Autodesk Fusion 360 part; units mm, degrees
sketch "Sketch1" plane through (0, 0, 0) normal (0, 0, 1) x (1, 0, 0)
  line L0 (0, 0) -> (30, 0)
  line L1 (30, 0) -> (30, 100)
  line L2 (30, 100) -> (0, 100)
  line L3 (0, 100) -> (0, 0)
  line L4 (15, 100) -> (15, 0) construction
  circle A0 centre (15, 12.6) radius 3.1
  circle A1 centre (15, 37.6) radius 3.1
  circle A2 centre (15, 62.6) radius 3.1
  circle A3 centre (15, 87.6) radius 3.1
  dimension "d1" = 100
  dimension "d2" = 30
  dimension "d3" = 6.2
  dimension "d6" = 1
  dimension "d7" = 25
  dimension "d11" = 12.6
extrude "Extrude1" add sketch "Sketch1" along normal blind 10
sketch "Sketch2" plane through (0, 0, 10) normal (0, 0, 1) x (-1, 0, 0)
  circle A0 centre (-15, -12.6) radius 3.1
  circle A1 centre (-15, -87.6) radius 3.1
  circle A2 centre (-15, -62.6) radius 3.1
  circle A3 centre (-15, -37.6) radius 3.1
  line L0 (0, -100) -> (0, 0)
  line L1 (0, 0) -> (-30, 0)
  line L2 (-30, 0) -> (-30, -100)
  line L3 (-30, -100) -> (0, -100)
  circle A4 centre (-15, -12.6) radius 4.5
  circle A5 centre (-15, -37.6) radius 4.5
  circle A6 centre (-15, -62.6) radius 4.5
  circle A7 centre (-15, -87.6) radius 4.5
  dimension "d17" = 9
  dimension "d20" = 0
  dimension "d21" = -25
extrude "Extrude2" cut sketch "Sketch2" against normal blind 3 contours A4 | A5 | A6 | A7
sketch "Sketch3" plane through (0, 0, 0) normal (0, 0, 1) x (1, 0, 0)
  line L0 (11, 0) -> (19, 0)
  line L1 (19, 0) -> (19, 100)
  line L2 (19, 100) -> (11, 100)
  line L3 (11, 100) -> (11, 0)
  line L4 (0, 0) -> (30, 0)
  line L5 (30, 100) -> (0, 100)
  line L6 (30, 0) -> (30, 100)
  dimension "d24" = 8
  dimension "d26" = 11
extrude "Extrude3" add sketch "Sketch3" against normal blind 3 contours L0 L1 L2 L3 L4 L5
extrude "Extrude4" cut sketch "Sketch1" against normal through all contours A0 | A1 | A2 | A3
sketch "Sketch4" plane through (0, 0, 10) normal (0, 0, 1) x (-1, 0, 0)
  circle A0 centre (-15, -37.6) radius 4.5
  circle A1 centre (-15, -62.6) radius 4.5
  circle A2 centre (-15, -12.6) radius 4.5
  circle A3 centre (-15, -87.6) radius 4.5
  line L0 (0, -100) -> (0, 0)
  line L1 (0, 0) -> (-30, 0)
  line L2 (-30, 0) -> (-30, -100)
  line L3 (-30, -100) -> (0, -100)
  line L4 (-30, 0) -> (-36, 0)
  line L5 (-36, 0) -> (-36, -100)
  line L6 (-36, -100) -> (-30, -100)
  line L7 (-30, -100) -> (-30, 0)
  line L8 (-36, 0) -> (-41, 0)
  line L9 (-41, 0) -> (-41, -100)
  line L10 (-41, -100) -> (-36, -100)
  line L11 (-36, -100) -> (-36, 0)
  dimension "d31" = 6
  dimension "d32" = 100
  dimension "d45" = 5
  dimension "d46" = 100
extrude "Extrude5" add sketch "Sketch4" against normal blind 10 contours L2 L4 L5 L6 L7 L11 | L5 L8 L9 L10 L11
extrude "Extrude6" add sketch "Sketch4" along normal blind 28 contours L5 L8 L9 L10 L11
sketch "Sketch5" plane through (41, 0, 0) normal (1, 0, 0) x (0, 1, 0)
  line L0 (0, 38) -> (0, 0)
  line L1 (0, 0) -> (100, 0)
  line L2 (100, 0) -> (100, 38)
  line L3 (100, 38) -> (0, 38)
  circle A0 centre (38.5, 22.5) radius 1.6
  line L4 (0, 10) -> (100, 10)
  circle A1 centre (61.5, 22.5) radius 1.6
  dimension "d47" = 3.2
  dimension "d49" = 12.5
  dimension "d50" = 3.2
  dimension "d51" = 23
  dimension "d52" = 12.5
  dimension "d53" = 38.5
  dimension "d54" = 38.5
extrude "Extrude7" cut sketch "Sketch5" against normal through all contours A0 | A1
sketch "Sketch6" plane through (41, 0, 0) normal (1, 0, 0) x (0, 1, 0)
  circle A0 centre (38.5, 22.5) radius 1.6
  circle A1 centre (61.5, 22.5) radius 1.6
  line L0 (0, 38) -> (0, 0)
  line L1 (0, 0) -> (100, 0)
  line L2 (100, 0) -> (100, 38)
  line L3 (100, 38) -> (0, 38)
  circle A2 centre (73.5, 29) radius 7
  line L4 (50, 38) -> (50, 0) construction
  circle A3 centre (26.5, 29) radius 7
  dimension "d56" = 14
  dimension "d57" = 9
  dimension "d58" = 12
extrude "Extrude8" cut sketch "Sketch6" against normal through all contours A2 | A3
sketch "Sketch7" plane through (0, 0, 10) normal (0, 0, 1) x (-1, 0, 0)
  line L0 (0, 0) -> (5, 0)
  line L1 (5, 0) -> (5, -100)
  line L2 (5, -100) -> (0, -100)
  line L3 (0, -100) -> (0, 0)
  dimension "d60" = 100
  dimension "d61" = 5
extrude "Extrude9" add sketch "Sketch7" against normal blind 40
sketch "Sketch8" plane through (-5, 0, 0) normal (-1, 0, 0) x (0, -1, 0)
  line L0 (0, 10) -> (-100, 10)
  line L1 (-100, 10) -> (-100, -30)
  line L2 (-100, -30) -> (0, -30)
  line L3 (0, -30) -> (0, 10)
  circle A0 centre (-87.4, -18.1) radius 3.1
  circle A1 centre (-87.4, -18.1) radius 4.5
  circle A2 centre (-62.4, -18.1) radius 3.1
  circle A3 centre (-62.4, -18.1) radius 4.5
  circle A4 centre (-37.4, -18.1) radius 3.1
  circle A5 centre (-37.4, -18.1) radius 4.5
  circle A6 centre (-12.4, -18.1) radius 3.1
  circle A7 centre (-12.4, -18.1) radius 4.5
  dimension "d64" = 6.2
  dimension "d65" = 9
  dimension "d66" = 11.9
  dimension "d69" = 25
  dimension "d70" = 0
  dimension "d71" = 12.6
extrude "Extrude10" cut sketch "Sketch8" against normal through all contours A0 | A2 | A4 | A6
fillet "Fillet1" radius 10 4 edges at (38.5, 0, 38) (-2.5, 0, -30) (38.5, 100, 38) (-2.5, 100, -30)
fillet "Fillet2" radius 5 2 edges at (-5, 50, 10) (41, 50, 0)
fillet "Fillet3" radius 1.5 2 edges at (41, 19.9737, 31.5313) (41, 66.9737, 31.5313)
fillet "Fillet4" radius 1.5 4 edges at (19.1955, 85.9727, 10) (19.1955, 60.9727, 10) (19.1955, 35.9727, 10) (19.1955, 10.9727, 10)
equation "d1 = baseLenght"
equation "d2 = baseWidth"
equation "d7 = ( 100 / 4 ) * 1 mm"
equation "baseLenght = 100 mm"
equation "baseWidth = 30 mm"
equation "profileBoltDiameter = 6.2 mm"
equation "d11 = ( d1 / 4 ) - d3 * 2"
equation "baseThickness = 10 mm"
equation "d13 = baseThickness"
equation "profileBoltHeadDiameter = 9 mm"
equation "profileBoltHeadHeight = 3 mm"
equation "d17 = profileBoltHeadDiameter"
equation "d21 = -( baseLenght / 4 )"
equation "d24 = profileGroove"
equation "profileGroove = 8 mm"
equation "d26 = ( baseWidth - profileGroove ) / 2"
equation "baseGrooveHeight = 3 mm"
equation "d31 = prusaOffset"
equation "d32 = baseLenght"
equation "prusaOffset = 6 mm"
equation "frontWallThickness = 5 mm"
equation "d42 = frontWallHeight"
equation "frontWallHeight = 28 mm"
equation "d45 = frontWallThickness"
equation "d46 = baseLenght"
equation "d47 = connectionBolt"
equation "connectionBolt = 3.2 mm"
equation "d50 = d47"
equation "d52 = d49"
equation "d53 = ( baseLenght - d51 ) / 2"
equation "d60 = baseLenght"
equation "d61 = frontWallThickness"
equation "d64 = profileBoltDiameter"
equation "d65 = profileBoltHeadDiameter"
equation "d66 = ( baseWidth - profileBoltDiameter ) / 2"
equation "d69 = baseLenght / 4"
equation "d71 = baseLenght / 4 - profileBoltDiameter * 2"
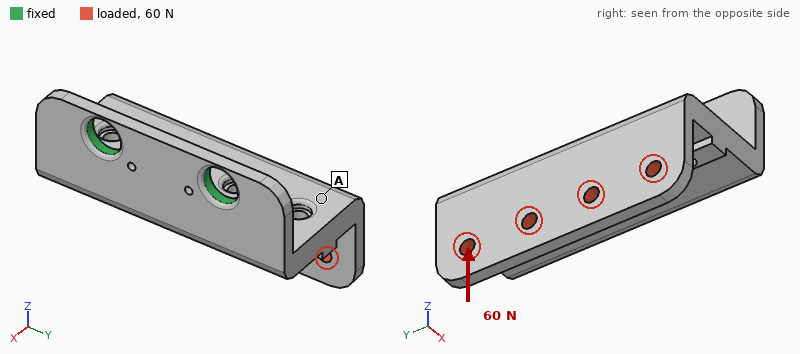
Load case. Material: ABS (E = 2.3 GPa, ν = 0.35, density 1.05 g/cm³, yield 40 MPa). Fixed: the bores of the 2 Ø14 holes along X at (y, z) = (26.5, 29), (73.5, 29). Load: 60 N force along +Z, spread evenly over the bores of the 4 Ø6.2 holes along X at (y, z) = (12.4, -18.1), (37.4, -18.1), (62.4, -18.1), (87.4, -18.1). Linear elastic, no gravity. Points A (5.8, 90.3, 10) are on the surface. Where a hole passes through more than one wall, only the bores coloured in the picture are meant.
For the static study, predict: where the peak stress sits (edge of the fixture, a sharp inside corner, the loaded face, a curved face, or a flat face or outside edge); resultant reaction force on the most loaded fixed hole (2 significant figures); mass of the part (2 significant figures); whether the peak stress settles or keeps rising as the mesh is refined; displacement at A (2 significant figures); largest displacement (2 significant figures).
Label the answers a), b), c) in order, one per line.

a) edge of the fixture
b) 30 N
c) 75 g
d) keeps rising
e) 0.66 mm
f) 1.3 mm
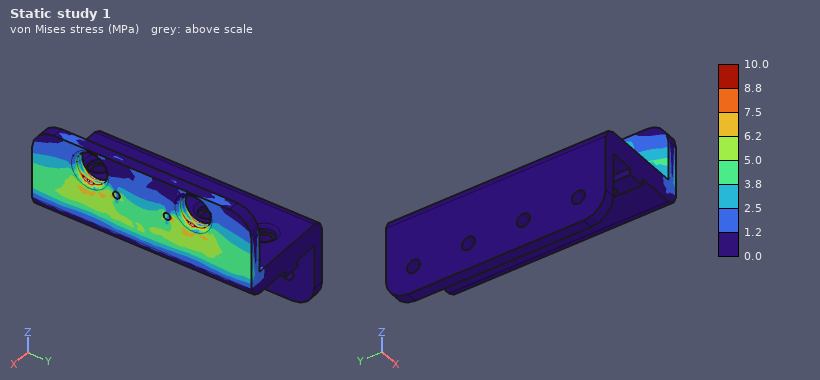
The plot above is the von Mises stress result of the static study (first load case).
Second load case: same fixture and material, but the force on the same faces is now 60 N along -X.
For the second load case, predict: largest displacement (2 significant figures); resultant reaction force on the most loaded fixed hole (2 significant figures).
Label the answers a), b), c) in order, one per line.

a) 1.3 mm
b) 30 N
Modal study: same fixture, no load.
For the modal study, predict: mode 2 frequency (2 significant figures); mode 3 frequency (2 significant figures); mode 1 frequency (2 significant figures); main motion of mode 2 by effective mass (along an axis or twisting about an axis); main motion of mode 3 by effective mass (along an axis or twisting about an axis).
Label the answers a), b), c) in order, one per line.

a) 560 Hz
b) 780 Hz
c) 200 Hz
d) along Y
e) along Y
